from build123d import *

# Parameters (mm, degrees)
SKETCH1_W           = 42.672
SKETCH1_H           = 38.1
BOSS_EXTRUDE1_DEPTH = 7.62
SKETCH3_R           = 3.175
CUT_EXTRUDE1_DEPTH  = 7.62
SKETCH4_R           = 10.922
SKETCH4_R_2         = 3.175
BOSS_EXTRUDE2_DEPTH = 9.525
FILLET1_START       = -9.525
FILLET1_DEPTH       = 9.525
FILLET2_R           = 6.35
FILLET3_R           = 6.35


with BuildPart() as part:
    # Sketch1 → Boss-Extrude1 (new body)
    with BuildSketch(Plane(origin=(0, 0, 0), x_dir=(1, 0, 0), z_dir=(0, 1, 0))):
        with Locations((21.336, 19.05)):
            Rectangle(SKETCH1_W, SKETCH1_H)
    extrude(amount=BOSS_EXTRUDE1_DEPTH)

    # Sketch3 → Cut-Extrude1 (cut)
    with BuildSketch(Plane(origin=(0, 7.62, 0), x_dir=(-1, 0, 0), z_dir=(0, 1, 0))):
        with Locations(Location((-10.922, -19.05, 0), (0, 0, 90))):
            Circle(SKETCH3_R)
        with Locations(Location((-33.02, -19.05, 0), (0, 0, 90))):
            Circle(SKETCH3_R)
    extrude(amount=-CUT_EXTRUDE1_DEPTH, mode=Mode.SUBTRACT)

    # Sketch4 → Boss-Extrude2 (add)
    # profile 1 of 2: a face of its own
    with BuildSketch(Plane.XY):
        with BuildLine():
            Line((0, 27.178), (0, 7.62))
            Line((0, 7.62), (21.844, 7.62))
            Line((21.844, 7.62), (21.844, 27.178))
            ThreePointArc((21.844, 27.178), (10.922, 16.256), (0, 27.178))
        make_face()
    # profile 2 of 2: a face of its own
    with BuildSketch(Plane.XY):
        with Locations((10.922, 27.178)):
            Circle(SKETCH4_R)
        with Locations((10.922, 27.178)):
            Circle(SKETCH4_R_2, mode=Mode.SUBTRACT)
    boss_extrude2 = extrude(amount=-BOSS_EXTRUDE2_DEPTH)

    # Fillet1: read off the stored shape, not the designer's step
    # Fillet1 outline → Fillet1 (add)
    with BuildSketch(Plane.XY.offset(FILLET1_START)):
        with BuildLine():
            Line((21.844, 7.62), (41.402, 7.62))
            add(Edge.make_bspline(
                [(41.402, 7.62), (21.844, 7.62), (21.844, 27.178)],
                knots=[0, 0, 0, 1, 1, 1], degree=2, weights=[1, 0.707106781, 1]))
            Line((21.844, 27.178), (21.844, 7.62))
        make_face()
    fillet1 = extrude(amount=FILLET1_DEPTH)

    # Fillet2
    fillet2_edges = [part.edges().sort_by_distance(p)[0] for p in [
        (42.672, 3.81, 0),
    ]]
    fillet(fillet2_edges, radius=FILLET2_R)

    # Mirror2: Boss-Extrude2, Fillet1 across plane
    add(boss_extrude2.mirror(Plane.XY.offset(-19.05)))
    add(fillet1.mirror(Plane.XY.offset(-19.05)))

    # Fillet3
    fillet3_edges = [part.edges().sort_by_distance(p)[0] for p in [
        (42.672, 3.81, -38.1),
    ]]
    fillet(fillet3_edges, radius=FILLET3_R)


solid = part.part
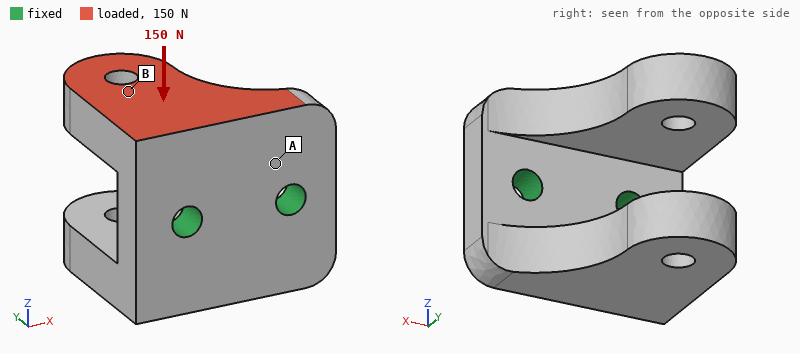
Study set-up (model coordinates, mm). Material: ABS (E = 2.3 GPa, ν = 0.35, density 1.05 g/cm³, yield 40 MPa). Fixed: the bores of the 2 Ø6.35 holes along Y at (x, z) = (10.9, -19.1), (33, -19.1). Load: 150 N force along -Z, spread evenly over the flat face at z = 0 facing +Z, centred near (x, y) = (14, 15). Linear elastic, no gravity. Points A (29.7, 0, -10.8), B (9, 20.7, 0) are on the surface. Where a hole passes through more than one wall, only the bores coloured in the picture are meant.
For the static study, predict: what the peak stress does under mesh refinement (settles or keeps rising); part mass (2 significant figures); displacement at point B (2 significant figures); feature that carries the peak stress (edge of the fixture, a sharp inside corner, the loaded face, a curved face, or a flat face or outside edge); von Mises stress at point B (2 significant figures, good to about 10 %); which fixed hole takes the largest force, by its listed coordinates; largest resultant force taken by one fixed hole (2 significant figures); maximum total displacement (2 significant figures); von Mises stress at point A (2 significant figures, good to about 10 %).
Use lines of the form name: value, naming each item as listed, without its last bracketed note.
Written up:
what the peak stress does under mesh refinement: keeps rising
part mass: 26 g
displacement at point B: 0.17 mm
feature that carries the peak stress: edge of the fixture
von Mises stress at point B: 1.0 MPa
which fixed hole takes the largest force, by its listed coordinates: (10.9, -19.1)
largest resultant force taken by one fixed hole: 120 N
maximum total displacement: 0.32 mm
von Mises stress at point A: 3.1 MPa
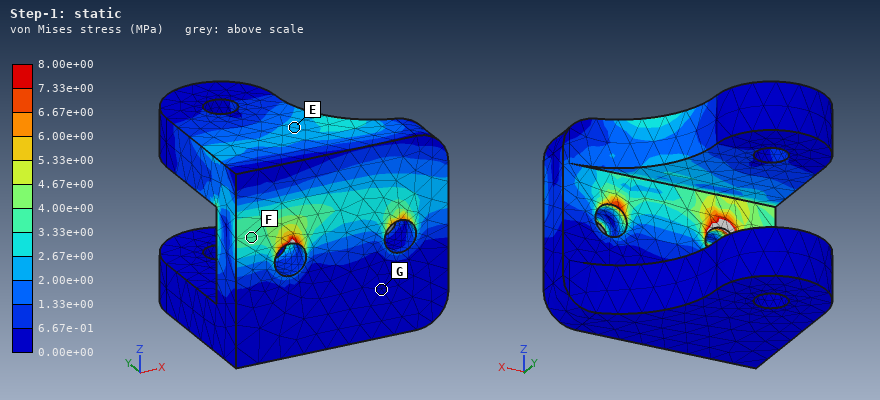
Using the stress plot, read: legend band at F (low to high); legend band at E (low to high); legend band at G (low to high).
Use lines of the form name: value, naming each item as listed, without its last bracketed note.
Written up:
legend band at F: 3.33e+00 to 4.00e+00 MPa
legend band at E: 2.00e+00 to 2.67e+00 MPa
legend band at G: 0.00e+00 to 6.67e-01 MPa
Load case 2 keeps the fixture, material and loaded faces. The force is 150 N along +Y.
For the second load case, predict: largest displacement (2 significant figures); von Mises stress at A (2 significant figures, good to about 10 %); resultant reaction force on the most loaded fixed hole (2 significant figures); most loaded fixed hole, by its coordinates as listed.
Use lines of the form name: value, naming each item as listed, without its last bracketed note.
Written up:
largest displacement: 0.30 mm
von Mises stress at A: 3.6 MPa
resultant reaction force on the most loaded fixed hole: 110 N
most loaded fixed hole, by its coordinates as listed: (10.9, -19.1)
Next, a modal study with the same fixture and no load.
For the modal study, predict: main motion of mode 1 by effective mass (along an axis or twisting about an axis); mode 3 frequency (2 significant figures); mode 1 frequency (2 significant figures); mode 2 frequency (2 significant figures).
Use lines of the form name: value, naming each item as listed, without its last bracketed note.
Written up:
main motion of mode 1 by effective mass: along Z
mode 3 frequency: 2500 Hz
mode 1 frequency: 1300 Hz
mode 2 frequency: 1400 Hz
